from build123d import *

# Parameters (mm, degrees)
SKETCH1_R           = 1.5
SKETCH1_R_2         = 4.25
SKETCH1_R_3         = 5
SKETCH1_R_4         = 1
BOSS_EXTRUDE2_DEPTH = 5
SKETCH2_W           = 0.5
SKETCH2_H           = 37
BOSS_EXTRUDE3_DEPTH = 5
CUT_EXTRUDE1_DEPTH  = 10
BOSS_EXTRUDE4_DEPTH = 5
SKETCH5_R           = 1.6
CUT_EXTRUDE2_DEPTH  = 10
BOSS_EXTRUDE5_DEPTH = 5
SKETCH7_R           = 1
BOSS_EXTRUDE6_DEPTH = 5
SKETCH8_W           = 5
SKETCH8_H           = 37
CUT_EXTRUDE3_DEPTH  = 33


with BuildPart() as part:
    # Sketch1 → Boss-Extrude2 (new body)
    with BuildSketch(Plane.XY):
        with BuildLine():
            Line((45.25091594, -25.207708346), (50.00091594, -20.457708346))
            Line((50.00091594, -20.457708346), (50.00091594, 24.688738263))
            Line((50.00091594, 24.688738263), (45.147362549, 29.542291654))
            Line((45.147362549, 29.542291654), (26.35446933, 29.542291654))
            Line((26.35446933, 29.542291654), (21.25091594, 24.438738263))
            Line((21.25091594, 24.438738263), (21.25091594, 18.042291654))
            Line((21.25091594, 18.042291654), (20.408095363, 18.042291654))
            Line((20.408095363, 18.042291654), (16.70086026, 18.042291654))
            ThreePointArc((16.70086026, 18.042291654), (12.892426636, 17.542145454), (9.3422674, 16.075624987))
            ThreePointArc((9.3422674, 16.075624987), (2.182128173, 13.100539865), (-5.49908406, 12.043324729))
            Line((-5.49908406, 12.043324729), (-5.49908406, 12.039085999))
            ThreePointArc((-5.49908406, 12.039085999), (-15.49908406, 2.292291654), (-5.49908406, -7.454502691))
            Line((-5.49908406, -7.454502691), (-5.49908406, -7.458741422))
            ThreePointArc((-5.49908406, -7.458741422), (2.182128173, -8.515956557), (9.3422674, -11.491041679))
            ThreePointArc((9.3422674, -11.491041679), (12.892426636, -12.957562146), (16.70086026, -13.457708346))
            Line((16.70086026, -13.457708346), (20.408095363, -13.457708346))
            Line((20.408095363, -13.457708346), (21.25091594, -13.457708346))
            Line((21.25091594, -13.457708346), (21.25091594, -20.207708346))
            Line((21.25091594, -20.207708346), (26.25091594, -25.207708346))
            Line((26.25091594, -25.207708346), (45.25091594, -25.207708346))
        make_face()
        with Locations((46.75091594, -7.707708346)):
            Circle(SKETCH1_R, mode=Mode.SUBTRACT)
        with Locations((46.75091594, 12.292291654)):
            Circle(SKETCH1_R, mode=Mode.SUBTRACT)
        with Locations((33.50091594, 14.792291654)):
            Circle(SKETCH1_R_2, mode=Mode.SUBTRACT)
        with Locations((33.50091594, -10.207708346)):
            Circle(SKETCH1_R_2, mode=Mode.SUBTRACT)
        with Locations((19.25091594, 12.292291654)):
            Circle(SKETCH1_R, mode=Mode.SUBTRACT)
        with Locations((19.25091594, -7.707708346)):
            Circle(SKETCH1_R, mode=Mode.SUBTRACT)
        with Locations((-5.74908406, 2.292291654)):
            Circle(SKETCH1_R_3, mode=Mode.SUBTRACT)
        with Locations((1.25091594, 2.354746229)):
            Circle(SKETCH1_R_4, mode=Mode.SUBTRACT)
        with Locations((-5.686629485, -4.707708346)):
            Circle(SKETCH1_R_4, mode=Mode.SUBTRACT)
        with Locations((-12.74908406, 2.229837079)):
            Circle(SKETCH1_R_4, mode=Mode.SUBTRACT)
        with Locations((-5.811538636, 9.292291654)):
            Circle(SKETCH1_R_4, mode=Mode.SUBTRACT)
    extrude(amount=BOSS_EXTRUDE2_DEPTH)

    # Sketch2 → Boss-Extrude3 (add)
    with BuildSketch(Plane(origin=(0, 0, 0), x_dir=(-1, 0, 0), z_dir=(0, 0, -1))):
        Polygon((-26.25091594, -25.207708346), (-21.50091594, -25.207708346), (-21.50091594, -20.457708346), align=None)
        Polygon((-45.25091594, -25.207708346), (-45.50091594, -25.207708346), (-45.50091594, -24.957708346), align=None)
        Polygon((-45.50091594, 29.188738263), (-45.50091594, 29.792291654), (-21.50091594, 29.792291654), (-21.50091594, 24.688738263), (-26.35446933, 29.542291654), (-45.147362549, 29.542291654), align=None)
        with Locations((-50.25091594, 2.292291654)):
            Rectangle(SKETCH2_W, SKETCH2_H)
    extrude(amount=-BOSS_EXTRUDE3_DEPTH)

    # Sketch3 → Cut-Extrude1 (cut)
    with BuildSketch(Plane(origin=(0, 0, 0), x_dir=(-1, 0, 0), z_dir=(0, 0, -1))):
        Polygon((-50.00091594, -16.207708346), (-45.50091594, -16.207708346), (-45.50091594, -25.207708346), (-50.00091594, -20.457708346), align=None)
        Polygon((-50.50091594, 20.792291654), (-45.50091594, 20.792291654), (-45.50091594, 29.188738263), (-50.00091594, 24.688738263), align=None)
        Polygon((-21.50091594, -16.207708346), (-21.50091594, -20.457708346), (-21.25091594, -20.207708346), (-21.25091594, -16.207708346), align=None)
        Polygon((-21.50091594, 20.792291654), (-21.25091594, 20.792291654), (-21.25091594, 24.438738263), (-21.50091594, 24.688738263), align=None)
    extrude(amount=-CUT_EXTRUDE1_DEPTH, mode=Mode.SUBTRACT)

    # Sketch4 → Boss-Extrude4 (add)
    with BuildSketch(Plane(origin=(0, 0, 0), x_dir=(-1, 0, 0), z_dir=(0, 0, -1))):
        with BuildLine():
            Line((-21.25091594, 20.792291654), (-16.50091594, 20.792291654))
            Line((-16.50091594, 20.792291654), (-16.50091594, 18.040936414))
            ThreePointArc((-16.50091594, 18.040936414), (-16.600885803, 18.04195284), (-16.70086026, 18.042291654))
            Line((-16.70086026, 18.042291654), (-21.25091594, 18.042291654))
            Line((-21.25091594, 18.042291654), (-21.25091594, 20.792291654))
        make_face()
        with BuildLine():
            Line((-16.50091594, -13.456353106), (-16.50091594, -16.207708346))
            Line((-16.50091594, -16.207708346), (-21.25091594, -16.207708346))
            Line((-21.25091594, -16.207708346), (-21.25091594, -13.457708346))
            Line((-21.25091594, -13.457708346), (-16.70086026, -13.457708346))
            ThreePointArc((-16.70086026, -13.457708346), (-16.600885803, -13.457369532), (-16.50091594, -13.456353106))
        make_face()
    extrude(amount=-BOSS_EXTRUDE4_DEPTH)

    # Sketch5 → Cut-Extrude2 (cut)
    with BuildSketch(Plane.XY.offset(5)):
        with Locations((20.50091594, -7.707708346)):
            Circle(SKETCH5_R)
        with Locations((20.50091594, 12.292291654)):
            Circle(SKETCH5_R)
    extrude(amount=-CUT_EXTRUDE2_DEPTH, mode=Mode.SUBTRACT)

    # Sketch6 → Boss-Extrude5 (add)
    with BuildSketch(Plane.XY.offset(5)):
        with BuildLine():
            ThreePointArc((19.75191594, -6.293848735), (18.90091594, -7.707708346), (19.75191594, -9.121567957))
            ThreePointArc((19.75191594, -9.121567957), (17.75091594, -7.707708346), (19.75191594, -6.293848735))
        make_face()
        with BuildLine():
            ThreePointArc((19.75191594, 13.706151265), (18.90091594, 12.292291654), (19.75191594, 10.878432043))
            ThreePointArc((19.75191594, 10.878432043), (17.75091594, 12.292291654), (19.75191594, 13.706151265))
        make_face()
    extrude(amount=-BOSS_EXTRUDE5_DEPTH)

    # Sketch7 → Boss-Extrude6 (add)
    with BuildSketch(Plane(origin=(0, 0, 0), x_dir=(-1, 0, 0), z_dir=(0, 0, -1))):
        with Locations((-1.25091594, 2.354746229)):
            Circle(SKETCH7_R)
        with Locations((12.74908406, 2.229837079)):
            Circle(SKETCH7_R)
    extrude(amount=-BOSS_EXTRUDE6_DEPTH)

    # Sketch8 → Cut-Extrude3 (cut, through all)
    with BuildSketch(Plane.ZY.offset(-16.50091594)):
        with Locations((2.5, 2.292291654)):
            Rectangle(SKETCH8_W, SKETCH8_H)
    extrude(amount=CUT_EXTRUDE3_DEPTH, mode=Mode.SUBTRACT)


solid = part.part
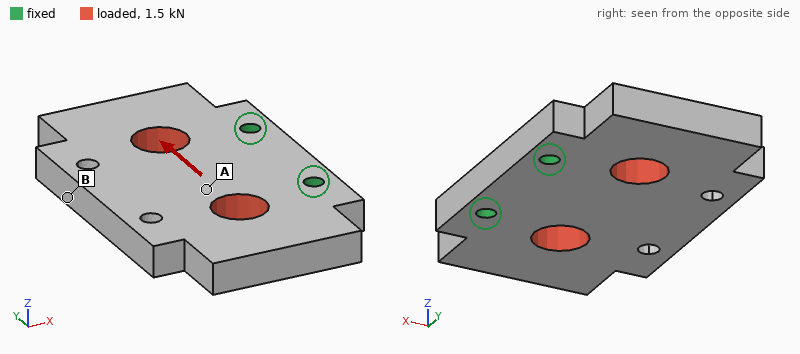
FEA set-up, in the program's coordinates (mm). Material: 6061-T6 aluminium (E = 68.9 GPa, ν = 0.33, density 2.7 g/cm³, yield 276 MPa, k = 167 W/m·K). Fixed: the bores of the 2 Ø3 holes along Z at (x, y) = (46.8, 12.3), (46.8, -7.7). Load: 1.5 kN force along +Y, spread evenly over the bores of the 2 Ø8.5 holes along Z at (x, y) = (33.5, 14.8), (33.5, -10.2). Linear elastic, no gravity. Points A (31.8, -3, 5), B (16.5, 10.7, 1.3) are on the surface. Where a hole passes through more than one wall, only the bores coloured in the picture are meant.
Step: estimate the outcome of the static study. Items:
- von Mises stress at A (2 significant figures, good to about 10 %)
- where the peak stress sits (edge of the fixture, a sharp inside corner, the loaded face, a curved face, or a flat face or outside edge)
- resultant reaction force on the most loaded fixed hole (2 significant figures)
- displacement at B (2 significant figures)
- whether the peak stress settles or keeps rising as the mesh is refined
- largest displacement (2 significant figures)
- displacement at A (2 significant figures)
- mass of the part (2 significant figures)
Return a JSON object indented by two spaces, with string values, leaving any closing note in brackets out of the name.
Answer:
{
  "von Mises stress at A": "17 MPa",
  "where the peak stress sits": "edge of the fixture",
  "resultant reaction force on the most loaded fixed hole": "1.1 kN",
  "displacement at B": "16 µm",
  "whether the peak stress settles or keeps rising as the mesh is refined": "keeps rising",
  "largest displacement": "17 µm",
  "displacement at A": "8.7 µm",
  "mass of the part": "21 g"
}
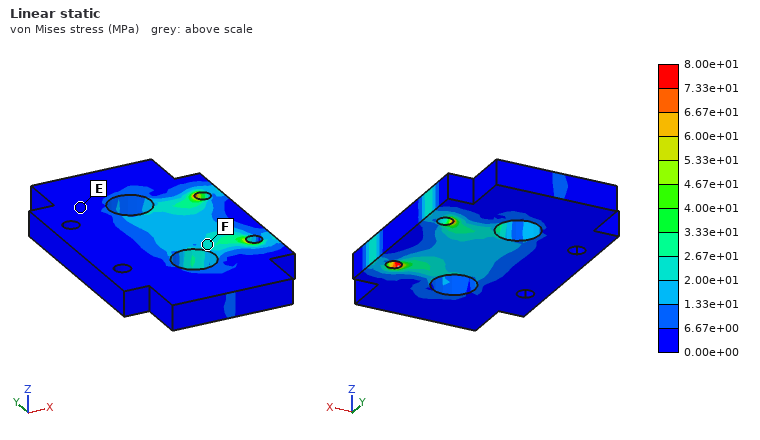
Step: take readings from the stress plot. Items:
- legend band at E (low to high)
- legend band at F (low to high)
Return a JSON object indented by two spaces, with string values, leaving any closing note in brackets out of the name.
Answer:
{
  "legend band at E": "0.00e+00 to 6.67e+00 MPa",
  "legend band at F": "2.00e+01 to 2.67e+01 MPa"
}
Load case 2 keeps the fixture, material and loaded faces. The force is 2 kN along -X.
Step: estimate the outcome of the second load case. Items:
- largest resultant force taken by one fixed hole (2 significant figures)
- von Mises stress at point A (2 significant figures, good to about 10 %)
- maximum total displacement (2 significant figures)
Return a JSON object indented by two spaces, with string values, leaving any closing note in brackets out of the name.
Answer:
{
  "largest resultant force taken by one fixed hole": "1.0 kN",
  "von Mises stress at point A": "6.7 MPa",
  "maximum total displacement": "5.2 µm"
}
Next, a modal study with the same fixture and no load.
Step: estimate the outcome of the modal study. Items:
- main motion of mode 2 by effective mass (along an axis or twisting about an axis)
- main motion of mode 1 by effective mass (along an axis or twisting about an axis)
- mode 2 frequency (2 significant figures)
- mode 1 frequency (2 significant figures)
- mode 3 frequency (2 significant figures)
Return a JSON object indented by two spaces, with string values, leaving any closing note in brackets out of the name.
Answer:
{
  "main motion of mode 2 by effective mass": "twisting about X",
  "main motion of mode 1 by effective mass": "along Z",
  "mode 2 frequency": "5500 Hz",
  "mode 1 frequency": "3700 Hz",
  "mode 3 frequency": "9500 Hz"
}
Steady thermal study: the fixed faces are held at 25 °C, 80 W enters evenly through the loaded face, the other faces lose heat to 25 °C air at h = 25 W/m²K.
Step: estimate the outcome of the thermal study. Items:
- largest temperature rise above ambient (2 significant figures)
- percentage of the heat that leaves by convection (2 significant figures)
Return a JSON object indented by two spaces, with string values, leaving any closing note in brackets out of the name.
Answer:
{
  "largest temperature rise above ambient": "44 K",
  "percentage of the heat that leaves by convection": "3.6 %"
}
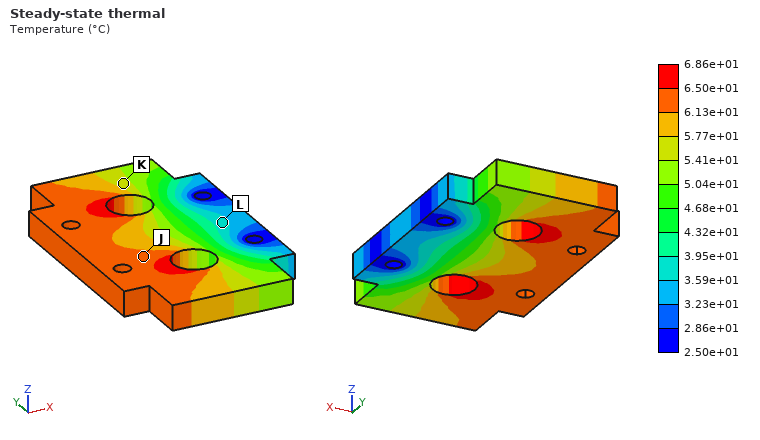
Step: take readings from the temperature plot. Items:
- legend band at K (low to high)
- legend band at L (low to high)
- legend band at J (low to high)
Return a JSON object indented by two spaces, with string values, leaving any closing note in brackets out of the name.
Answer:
{
  "legend band at K": "5.41e+01 to 5.77e+01 °C",
  "legend band at L": "3.59e+01 to 3.95e+01 °C",
  "legend band at J": "6.13e+01 to 6.50e+01 °C"
}
